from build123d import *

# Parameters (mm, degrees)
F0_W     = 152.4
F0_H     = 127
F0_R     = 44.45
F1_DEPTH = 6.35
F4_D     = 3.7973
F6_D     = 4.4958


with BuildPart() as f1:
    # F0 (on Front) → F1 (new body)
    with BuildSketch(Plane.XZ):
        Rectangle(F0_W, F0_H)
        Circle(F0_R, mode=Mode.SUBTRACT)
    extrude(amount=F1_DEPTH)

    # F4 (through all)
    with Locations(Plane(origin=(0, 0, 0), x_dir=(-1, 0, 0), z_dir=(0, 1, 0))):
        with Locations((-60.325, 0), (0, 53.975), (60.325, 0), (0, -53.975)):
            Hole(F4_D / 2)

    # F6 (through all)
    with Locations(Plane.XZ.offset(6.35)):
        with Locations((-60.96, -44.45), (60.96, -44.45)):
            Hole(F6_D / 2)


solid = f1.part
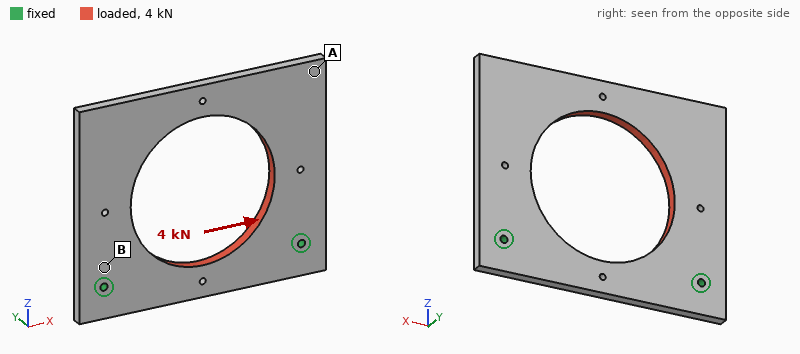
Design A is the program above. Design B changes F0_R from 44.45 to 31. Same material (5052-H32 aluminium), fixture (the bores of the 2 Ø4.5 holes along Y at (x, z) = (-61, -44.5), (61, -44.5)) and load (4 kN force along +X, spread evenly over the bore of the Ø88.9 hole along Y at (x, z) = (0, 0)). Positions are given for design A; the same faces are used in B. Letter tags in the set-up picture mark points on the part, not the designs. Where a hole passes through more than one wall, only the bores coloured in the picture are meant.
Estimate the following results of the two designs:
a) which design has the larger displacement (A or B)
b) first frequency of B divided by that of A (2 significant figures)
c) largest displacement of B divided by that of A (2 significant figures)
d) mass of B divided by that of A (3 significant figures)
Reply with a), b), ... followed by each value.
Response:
a) A
b) 1.0
c) 0.38
d) 1.24
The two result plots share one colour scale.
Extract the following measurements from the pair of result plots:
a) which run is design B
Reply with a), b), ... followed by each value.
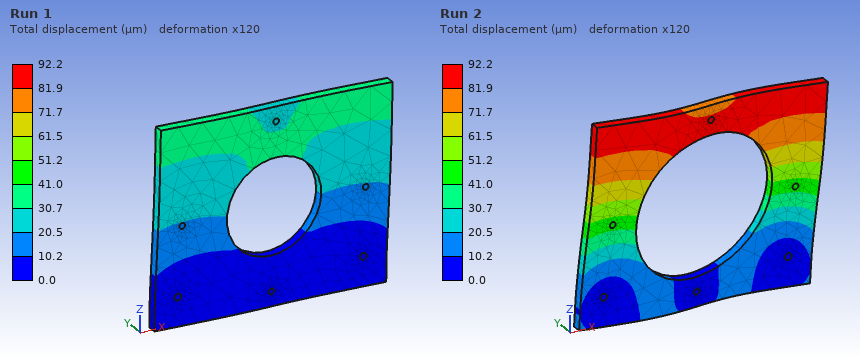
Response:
a) Run 1
